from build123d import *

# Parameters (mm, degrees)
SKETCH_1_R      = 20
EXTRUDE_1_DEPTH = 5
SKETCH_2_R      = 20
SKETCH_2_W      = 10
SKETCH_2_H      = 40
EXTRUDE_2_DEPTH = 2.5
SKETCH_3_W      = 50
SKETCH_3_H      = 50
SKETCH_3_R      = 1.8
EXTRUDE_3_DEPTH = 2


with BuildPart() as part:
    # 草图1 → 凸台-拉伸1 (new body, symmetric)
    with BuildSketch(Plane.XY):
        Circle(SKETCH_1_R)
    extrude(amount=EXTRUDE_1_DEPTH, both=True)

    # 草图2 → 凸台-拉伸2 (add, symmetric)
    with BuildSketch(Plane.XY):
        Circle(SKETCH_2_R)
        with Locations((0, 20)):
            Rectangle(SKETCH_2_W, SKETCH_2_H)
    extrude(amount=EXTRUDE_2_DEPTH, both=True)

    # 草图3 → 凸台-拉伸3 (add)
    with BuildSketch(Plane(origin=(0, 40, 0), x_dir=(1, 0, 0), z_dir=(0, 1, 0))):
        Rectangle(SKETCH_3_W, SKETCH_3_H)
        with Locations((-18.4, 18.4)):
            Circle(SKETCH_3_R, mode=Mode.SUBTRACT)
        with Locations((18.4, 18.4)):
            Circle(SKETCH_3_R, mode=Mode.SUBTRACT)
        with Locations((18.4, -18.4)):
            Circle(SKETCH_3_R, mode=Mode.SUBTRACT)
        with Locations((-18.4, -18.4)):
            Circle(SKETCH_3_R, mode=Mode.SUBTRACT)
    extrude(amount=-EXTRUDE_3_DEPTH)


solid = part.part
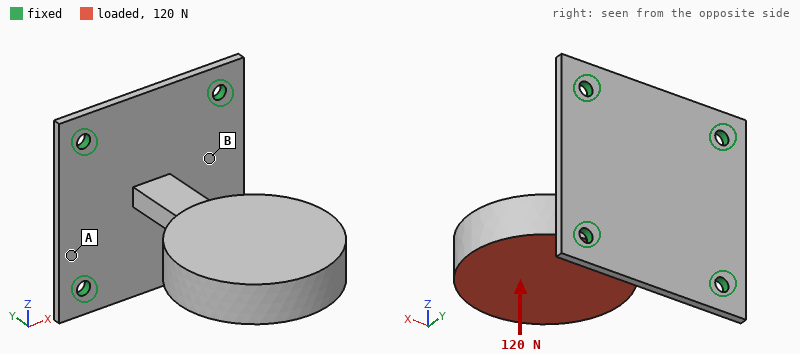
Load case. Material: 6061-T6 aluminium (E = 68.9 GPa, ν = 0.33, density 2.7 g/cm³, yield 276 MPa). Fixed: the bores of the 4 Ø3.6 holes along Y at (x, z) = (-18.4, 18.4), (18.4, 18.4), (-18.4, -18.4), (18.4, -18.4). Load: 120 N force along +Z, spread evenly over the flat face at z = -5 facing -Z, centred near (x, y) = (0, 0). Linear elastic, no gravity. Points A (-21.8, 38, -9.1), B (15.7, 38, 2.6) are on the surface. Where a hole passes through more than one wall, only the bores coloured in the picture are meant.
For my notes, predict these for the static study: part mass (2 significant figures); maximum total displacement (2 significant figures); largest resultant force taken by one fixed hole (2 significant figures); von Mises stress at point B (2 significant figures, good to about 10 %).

50 g
1.1 mm
86 N
30 MPa
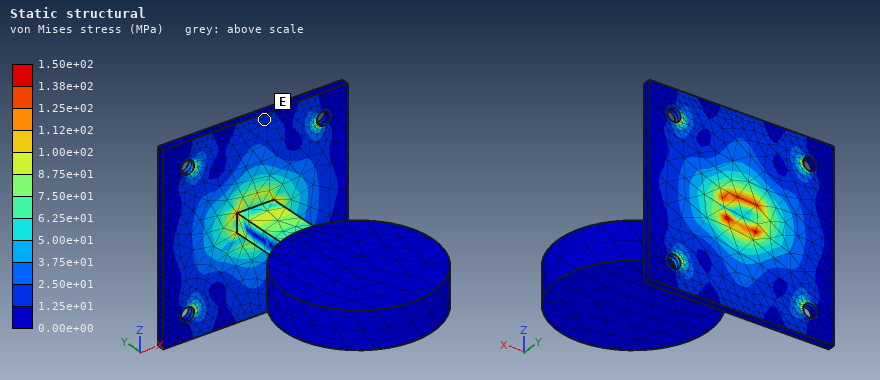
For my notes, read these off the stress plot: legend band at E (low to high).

1.25e+01 to 2.50e+01 MPa
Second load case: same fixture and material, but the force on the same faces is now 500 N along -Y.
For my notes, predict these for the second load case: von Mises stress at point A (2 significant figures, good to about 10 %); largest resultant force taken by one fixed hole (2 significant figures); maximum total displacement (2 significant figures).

31 MPa
170 N
0.67 mm
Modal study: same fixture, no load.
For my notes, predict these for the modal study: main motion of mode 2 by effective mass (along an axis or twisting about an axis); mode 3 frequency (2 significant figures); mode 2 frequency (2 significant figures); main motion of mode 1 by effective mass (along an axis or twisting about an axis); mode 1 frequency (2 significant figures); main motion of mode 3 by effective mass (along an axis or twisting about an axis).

along X
1600 Hz
460 Hz
along Z
350 Hz
along Y
